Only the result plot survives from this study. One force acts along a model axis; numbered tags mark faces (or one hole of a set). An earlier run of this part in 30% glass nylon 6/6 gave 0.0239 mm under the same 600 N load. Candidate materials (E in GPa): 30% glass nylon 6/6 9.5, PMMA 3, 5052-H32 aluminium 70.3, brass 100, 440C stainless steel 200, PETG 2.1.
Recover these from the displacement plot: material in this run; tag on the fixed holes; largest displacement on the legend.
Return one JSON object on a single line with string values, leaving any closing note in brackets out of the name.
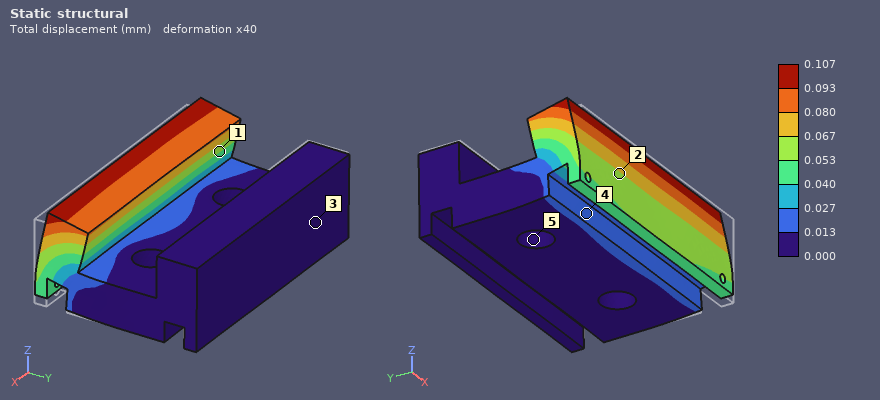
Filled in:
{"material in this run": "PETG", "tag on the fixed holes": "5", "largest displacement on the legend": "0.107 mm"}
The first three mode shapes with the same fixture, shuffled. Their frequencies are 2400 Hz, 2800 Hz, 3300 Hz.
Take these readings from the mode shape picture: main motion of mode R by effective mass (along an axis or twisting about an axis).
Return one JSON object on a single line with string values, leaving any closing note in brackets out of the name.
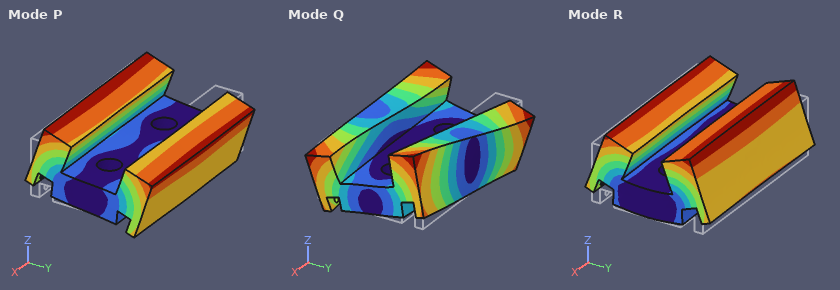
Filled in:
{"main motion of mode R by effective mass": "along Z"}
